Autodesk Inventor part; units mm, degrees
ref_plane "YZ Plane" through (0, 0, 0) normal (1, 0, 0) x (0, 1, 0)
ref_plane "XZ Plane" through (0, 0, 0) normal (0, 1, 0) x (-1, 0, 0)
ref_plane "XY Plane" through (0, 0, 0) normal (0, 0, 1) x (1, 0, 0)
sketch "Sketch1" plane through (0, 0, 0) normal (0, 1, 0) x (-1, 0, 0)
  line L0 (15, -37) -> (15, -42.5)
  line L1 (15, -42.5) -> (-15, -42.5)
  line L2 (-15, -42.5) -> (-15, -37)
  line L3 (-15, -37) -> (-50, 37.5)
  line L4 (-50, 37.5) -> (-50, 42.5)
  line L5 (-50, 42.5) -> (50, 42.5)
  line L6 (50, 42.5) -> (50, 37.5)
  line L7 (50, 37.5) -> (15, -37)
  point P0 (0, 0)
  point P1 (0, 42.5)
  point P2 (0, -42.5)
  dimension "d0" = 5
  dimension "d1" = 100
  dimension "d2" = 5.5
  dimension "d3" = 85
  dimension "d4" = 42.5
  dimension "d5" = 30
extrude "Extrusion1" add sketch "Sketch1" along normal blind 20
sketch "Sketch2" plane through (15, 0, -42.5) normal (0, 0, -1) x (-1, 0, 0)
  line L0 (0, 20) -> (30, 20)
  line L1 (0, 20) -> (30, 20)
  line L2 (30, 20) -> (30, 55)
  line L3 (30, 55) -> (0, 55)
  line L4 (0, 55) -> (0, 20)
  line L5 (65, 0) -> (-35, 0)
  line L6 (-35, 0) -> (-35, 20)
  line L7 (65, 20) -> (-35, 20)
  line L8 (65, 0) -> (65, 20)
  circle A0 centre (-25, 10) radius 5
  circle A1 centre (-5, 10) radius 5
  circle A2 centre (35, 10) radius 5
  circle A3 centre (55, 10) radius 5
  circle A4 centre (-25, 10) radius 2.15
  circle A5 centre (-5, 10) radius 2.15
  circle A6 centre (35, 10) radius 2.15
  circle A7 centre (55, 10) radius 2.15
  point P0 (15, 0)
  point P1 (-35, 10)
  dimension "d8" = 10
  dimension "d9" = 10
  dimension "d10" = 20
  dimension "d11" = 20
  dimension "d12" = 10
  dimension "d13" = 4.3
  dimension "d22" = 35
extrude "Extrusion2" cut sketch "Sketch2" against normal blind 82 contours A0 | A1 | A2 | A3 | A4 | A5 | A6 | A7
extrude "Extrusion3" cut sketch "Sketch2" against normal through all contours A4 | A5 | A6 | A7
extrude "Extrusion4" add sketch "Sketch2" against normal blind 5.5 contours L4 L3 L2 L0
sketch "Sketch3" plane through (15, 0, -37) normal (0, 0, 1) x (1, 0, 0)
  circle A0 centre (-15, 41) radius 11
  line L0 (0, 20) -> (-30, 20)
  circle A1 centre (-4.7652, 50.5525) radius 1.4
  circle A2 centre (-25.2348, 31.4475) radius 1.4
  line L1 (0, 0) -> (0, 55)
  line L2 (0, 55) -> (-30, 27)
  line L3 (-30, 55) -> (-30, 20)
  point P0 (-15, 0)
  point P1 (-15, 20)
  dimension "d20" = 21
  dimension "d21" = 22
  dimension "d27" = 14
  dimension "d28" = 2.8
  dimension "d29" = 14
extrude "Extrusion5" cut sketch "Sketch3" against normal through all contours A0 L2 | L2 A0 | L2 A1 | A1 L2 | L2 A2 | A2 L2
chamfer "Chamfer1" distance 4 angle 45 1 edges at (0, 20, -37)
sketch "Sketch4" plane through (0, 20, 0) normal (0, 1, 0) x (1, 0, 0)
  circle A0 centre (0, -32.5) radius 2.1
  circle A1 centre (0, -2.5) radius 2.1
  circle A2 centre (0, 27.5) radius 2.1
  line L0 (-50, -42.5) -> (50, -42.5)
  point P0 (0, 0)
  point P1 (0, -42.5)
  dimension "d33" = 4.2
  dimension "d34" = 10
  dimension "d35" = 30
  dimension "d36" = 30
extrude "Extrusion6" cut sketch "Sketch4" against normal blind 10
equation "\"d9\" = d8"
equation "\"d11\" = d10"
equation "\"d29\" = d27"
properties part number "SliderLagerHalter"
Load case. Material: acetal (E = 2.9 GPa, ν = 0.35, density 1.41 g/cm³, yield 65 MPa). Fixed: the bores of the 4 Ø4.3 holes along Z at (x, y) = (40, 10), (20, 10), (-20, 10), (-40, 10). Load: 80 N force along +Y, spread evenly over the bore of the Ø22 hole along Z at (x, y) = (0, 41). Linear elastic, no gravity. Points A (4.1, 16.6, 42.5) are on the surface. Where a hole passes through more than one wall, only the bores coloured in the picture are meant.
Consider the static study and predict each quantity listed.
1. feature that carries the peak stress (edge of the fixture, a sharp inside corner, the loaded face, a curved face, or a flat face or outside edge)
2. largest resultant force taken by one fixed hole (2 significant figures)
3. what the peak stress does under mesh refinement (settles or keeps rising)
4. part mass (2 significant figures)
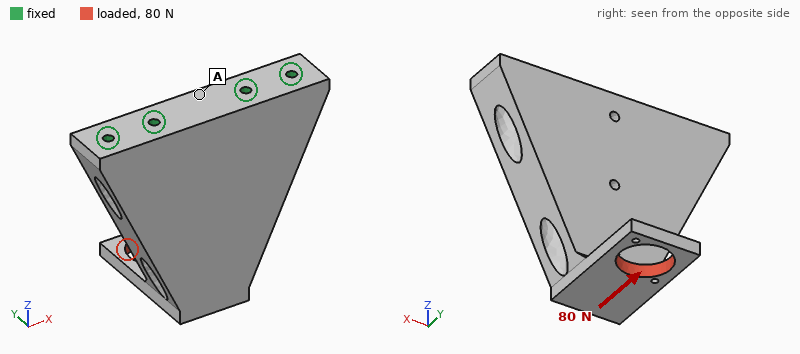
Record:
edge of the fixture
39 N
keeps rising
140 g
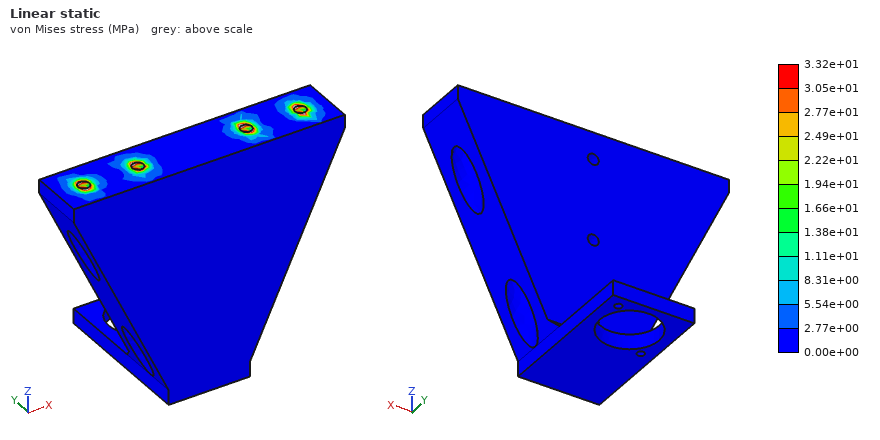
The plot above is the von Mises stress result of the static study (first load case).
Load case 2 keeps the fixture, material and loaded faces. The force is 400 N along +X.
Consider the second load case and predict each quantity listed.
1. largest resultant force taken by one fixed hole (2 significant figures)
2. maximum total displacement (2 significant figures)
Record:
360 N
1.3 mm
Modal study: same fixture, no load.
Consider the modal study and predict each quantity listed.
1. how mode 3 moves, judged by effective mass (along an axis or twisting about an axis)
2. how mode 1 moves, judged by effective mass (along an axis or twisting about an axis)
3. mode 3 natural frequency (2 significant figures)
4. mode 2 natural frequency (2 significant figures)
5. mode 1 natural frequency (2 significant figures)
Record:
along X
along Y
1300 Hz
980 Hz
200 Hz
